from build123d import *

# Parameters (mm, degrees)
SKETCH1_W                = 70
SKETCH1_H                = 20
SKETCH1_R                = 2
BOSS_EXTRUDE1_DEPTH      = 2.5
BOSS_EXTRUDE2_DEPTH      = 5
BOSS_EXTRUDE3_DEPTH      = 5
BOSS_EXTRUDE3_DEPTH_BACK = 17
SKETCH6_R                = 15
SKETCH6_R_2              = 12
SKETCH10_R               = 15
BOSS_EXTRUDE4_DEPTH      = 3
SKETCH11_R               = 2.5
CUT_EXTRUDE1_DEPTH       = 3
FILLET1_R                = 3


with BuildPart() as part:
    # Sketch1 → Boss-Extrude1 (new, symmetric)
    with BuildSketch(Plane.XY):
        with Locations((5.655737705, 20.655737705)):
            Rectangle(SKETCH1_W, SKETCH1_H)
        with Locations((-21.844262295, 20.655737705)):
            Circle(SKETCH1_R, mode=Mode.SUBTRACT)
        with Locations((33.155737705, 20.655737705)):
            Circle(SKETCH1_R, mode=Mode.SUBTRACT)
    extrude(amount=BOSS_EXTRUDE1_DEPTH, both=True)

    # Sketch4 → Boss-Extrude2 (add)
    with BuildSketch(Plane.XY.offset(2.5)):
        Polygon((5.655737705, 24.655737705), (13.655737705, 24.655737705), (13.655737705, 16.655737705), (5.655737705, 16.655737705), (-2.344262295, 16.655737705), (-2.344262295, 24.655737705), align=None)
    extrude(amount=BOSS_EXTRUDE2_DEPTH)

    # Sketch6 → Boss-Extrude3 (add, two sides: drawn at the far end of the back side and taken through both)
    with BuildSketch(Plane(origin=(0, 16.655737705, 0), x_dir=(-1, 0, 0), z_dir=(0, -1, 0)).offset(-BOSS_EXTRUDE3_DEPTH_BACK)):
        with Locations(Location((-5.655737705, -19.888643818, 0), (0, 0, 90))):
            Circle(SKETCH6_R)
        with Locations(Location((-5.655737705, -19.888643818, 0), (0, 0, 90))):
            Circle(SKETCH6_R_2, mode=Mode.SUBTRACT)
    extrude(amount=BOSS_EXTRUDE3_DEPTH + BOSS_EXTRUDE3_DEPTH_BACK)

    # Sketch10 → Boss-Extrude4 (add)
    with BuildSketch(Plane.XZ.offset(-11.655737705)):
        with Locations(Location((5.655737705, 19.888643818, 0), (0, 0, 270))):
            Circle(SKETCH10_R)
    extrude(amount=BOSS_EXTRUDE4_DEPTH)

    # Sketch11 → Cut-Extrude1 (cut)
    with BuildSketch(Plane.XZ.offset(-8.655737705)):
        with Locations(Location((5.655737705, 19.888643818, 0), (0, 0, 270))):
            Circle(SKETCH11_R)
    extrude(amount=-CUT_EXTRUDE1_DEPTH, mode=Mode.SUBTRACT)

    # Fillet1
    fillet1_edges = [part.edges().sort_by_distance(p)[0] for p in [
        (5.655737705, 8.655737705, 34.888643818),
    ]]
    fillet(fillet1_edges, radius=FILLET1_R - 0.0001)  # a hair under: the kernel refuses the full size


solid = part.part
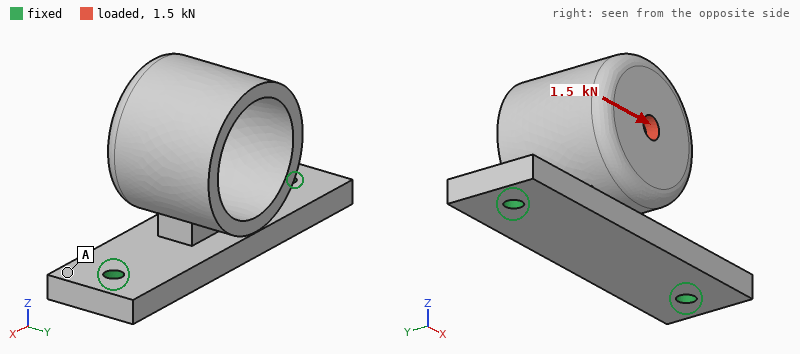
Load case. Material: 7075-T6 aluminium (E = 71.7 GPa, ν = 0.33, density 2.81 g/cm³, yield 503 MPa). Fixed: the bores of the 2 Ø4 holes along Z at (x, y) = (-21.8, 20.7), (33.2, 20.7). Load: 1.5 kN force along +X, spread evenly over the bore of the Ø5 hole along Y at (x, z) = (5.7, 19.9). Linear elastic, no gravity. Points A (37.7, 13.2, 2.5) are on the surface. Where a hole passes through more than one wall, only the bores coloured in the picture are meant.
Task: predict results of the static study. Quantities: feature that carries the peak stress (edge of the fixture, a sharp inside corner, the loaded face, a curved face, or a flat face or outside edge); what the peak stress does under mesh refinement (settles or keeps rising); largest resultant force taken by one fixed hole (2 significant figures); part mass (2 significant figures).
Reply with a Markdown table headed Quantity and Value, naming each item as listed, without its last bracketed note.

| Quantity | Value |
|---|---|
| feature that carries the peak stress | edge of the fixture |
| what the peak stress does under mesh refinement | keeps rising |
| largest resultant force taken by one fixed hole | 1.1 kN |
| part mass | 41 g |
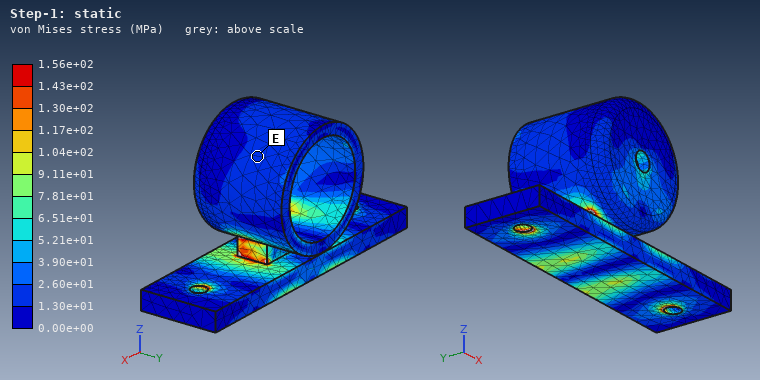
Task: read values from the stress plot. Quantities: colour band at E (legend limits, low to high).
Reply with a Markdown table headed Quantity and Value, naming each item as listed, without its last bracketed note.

| Quantity | Value |
|---|---|
| colour band at E | 1.30e+01 to 2.60e+01 MPa |
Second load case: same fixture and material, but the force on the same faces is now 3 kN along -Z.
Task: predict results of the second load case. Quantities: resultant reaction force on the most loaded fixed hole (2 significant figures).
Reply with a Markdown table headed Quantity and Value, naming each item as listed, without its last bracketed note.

| Quantity | Value |
|---|---|
| resultant reaction force on the most loaded fixed hole | 1.6 kN |
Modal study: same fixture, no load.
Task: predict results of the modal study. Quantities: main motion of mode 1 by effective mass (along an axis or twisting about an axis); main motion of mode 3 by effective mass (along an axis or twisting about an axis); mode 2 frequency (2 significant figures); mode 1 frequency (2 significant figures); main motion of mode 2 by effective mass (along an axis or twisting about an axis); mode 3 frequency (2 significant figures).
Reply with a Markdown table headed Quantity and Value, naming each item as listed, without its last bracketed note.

| Quantity | Value |
|---|---|
| main motion of mode 1 by effective mass | along Y |
| main motion of mode 3 by effective mass | along Z |
| mode 2 frequency | 2800 Hz |
| mode 1 frequency | 1700 Hz |
| main motion of mode 2 by effective mass | along X |
| mode 3 frequency | 4400 Hz |
